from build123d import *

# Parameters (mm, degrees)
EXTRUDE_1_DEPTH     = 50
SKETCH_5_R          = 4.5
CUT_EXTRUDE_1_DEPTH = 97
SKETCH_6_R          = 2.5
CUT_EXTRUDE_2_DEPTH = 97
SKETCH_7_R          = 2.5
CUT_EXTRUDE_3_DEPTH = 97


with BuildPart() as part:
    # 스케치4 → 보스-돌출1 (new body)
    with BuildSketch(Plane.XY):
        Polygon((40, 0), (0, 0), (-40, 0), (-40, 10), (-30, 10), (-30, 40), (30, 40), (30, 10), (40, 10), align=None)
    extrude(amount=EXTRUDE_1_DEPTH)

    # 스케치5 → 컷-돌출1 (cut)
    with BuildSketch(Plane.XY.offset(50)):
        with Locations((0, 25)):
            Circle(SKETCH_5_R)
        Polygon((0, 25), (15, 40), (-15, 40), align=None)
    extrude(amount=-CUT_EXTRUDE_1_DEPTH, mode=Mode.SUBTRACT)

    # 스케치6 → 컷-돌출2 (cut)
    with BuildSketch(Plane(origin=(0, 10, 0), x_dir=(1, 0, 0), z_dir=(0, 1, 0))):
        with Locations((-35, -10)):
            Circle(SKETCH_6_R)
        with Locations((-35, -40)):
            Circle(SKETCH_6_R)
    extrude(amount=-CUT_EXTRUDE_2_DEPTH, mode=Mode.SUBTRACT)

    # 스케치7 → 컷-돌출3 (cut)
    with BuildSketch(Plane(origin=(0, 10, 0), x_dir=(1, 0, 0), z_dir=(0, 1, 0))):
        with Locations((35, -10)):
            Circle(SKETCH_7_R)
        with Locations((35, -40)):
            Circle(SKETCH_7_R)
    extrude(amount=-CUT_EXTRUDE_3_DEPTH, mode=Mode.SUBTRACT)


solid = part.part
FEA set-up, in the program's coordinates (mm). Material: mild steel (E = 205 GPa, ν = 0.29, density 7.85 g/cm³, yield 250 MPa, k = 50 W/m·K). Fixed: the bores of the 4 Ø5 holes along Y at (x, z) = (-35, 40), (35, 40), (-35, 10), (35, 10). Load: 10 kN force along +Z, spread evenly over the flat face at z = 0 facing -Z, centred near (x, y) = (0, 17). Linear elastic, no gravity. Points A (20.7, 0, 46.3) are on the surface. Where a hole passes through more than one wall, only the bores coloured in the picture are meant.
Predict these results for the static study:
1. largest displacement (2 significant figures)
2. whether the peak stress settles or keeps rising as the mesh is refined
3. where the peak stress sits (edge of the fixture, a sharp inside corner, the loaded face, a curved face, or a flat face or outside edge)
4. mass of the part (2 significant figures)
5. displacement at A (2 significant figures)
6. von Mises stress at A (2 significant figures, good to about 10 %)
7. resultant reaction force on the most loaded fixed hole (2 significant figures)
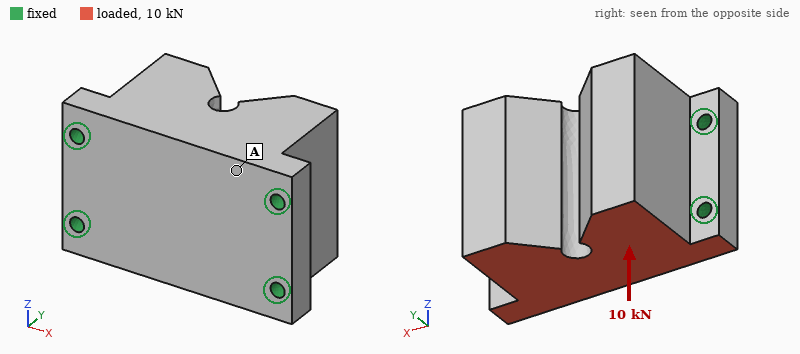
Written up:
7.6 µm
keeps rising
edge of the fixture
910 g
2.5 µm
9.8 MPa
3.5 kN
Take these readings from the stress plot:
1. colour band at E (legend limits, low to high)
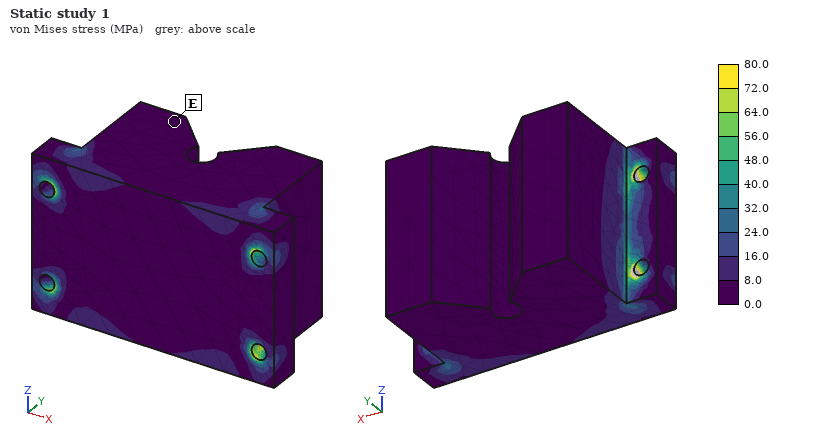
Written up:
0.0 to 8.0 MPa
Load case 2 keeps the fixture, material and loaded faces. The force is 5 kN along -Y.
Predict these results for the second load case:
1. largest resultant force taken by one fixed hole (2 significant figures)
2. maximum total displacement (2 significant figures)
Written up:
3.2 kN
7.1 µm
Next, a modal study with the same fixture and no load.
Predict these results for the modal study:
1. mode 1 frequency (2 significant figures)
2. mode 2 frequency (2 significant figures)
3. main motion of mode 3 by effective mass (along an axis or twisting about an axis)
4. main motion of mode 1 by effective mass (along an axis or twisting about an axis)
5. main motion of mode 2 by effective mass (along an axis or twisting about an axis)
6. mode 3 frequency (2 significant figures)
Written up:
7000 Hz
8600 Hz
along X
along Z
along Y
12 kHz
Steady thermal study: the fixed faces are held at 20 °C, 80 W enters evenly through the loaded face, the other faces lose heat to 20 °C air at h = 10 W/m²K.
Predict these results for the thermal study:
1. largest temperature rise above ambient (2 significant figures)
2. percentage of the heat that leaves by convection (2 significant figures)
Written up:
36 K
3.5 %
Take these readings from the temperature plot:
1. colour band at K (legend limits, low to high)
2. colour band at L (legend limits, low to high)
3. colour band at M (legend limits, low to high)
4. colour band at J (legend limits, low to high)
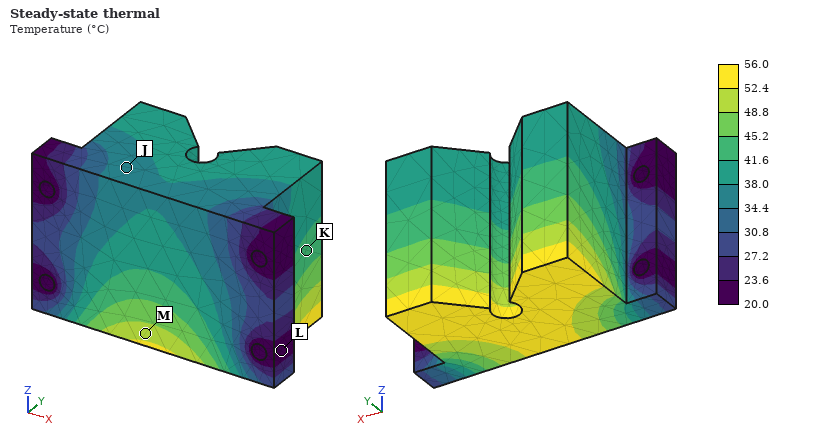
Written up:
41.6 to 45.2 °C
20.0 to 23.6 °C
48.8 to 52.4 °C
34.4 to 38.0 °C
